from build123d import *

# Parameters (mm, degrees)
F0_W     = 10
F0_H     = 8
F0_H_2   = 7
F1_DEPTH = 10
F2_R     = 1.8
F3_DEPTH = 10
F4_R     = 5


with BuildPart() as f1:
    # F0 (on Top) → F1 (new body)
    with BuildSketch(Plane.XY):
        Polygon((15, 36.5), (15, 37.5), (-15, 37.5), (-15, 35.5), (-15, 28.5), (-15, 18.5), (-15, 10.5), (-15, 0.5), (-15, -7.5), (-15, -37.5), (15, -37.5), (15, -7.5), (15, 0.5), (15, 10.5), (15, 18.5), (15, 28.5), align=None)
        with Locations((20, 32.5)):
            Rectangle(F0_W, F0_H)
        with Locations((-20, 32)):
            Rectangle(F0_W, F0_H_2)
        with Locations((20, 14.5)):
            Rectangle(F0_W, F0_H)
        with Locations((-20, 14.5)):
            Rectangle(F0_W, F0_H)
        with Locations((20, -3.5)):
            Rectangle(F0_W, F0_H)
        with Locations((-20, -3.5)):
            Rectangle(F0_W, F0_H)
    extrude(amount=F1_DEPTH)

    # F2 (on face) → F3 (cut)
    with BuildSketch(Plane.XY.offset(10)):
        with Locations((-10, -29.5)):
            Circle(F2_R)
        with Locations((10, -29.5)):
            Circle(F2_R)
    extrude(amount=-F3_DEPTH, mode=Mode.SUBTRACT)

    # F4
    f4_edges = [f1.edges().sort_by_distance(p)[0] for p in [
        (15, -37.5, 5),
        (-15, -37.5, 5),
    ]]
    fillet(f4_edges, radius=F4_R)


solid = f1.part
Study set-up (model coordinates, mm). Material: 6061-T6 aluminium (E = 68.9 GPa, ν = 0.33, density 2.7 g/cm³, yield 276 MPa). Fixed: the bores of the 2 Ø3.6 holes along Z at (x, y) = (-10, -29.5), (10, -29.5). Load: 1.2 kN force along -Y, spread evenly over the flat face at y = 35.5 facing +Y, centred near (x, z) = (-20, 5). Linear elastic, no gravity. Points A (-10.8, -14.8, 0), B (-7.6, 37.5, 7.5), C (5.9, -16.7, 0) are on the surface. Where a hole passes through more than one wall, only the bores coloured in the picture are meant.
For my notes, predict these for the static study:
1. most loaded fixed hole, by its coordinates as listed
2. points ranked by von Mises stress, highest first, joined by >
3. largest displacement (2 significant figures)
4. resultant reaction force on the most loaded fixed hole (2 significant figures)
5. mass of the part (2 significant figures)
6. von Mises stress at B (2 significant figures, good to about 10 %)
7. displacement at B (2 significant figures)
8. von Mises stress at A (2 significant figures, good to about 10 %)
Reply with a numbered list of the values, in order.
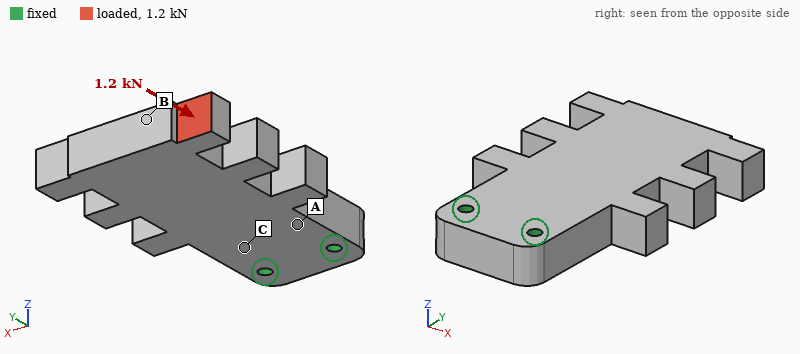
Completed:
1. (-10, -29.5)
2. B > A > C
3. 65 µm
4. 1.7 kN
5. 73 g
6. 28 MPa
7. 38 µm
8. 16 MPa
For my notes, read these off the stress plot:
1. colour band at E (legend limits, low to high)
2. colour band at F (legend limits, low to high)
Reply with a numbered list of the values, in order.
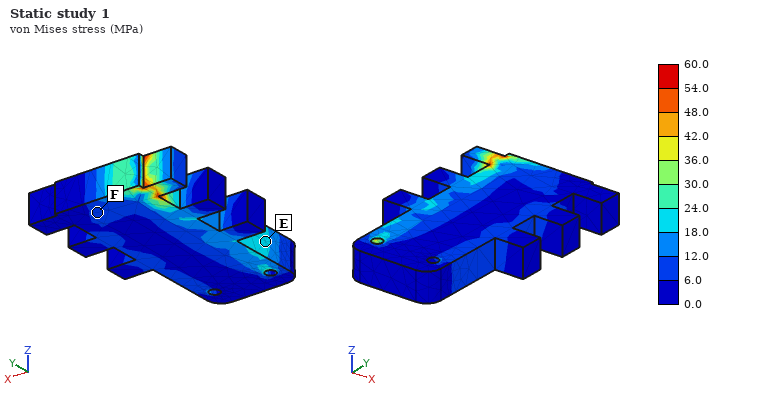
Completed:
1. 18.0 to 24.0 MPa
2. 6.0 to 12.0 MPa
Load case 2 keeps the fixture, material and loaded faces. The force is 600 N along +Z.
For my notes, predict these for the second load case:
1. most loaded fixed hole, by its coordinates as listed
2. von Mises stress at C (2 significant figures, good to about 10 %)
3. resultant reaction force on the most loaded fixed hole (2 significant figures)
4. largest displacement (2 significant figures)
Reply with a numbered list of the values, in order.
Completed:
1. (-10, -29.5)
2. 61 MPa
3. 780 N
4. 0.43 mm
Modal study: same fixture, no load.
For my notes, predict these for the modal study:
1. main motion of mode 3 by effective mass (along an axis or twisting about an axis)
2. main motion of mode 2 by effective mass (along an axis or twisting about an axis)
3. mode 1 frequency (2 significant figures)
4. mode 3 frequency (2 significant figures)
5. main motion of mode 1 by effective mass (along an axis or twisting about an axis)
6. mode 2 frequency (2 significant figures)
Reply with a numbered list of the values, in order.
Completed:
1. twisting about Y
2. along X
3. 1500 Hz
4. 4500 Hz
5. along Z
6. 4000 Hz
